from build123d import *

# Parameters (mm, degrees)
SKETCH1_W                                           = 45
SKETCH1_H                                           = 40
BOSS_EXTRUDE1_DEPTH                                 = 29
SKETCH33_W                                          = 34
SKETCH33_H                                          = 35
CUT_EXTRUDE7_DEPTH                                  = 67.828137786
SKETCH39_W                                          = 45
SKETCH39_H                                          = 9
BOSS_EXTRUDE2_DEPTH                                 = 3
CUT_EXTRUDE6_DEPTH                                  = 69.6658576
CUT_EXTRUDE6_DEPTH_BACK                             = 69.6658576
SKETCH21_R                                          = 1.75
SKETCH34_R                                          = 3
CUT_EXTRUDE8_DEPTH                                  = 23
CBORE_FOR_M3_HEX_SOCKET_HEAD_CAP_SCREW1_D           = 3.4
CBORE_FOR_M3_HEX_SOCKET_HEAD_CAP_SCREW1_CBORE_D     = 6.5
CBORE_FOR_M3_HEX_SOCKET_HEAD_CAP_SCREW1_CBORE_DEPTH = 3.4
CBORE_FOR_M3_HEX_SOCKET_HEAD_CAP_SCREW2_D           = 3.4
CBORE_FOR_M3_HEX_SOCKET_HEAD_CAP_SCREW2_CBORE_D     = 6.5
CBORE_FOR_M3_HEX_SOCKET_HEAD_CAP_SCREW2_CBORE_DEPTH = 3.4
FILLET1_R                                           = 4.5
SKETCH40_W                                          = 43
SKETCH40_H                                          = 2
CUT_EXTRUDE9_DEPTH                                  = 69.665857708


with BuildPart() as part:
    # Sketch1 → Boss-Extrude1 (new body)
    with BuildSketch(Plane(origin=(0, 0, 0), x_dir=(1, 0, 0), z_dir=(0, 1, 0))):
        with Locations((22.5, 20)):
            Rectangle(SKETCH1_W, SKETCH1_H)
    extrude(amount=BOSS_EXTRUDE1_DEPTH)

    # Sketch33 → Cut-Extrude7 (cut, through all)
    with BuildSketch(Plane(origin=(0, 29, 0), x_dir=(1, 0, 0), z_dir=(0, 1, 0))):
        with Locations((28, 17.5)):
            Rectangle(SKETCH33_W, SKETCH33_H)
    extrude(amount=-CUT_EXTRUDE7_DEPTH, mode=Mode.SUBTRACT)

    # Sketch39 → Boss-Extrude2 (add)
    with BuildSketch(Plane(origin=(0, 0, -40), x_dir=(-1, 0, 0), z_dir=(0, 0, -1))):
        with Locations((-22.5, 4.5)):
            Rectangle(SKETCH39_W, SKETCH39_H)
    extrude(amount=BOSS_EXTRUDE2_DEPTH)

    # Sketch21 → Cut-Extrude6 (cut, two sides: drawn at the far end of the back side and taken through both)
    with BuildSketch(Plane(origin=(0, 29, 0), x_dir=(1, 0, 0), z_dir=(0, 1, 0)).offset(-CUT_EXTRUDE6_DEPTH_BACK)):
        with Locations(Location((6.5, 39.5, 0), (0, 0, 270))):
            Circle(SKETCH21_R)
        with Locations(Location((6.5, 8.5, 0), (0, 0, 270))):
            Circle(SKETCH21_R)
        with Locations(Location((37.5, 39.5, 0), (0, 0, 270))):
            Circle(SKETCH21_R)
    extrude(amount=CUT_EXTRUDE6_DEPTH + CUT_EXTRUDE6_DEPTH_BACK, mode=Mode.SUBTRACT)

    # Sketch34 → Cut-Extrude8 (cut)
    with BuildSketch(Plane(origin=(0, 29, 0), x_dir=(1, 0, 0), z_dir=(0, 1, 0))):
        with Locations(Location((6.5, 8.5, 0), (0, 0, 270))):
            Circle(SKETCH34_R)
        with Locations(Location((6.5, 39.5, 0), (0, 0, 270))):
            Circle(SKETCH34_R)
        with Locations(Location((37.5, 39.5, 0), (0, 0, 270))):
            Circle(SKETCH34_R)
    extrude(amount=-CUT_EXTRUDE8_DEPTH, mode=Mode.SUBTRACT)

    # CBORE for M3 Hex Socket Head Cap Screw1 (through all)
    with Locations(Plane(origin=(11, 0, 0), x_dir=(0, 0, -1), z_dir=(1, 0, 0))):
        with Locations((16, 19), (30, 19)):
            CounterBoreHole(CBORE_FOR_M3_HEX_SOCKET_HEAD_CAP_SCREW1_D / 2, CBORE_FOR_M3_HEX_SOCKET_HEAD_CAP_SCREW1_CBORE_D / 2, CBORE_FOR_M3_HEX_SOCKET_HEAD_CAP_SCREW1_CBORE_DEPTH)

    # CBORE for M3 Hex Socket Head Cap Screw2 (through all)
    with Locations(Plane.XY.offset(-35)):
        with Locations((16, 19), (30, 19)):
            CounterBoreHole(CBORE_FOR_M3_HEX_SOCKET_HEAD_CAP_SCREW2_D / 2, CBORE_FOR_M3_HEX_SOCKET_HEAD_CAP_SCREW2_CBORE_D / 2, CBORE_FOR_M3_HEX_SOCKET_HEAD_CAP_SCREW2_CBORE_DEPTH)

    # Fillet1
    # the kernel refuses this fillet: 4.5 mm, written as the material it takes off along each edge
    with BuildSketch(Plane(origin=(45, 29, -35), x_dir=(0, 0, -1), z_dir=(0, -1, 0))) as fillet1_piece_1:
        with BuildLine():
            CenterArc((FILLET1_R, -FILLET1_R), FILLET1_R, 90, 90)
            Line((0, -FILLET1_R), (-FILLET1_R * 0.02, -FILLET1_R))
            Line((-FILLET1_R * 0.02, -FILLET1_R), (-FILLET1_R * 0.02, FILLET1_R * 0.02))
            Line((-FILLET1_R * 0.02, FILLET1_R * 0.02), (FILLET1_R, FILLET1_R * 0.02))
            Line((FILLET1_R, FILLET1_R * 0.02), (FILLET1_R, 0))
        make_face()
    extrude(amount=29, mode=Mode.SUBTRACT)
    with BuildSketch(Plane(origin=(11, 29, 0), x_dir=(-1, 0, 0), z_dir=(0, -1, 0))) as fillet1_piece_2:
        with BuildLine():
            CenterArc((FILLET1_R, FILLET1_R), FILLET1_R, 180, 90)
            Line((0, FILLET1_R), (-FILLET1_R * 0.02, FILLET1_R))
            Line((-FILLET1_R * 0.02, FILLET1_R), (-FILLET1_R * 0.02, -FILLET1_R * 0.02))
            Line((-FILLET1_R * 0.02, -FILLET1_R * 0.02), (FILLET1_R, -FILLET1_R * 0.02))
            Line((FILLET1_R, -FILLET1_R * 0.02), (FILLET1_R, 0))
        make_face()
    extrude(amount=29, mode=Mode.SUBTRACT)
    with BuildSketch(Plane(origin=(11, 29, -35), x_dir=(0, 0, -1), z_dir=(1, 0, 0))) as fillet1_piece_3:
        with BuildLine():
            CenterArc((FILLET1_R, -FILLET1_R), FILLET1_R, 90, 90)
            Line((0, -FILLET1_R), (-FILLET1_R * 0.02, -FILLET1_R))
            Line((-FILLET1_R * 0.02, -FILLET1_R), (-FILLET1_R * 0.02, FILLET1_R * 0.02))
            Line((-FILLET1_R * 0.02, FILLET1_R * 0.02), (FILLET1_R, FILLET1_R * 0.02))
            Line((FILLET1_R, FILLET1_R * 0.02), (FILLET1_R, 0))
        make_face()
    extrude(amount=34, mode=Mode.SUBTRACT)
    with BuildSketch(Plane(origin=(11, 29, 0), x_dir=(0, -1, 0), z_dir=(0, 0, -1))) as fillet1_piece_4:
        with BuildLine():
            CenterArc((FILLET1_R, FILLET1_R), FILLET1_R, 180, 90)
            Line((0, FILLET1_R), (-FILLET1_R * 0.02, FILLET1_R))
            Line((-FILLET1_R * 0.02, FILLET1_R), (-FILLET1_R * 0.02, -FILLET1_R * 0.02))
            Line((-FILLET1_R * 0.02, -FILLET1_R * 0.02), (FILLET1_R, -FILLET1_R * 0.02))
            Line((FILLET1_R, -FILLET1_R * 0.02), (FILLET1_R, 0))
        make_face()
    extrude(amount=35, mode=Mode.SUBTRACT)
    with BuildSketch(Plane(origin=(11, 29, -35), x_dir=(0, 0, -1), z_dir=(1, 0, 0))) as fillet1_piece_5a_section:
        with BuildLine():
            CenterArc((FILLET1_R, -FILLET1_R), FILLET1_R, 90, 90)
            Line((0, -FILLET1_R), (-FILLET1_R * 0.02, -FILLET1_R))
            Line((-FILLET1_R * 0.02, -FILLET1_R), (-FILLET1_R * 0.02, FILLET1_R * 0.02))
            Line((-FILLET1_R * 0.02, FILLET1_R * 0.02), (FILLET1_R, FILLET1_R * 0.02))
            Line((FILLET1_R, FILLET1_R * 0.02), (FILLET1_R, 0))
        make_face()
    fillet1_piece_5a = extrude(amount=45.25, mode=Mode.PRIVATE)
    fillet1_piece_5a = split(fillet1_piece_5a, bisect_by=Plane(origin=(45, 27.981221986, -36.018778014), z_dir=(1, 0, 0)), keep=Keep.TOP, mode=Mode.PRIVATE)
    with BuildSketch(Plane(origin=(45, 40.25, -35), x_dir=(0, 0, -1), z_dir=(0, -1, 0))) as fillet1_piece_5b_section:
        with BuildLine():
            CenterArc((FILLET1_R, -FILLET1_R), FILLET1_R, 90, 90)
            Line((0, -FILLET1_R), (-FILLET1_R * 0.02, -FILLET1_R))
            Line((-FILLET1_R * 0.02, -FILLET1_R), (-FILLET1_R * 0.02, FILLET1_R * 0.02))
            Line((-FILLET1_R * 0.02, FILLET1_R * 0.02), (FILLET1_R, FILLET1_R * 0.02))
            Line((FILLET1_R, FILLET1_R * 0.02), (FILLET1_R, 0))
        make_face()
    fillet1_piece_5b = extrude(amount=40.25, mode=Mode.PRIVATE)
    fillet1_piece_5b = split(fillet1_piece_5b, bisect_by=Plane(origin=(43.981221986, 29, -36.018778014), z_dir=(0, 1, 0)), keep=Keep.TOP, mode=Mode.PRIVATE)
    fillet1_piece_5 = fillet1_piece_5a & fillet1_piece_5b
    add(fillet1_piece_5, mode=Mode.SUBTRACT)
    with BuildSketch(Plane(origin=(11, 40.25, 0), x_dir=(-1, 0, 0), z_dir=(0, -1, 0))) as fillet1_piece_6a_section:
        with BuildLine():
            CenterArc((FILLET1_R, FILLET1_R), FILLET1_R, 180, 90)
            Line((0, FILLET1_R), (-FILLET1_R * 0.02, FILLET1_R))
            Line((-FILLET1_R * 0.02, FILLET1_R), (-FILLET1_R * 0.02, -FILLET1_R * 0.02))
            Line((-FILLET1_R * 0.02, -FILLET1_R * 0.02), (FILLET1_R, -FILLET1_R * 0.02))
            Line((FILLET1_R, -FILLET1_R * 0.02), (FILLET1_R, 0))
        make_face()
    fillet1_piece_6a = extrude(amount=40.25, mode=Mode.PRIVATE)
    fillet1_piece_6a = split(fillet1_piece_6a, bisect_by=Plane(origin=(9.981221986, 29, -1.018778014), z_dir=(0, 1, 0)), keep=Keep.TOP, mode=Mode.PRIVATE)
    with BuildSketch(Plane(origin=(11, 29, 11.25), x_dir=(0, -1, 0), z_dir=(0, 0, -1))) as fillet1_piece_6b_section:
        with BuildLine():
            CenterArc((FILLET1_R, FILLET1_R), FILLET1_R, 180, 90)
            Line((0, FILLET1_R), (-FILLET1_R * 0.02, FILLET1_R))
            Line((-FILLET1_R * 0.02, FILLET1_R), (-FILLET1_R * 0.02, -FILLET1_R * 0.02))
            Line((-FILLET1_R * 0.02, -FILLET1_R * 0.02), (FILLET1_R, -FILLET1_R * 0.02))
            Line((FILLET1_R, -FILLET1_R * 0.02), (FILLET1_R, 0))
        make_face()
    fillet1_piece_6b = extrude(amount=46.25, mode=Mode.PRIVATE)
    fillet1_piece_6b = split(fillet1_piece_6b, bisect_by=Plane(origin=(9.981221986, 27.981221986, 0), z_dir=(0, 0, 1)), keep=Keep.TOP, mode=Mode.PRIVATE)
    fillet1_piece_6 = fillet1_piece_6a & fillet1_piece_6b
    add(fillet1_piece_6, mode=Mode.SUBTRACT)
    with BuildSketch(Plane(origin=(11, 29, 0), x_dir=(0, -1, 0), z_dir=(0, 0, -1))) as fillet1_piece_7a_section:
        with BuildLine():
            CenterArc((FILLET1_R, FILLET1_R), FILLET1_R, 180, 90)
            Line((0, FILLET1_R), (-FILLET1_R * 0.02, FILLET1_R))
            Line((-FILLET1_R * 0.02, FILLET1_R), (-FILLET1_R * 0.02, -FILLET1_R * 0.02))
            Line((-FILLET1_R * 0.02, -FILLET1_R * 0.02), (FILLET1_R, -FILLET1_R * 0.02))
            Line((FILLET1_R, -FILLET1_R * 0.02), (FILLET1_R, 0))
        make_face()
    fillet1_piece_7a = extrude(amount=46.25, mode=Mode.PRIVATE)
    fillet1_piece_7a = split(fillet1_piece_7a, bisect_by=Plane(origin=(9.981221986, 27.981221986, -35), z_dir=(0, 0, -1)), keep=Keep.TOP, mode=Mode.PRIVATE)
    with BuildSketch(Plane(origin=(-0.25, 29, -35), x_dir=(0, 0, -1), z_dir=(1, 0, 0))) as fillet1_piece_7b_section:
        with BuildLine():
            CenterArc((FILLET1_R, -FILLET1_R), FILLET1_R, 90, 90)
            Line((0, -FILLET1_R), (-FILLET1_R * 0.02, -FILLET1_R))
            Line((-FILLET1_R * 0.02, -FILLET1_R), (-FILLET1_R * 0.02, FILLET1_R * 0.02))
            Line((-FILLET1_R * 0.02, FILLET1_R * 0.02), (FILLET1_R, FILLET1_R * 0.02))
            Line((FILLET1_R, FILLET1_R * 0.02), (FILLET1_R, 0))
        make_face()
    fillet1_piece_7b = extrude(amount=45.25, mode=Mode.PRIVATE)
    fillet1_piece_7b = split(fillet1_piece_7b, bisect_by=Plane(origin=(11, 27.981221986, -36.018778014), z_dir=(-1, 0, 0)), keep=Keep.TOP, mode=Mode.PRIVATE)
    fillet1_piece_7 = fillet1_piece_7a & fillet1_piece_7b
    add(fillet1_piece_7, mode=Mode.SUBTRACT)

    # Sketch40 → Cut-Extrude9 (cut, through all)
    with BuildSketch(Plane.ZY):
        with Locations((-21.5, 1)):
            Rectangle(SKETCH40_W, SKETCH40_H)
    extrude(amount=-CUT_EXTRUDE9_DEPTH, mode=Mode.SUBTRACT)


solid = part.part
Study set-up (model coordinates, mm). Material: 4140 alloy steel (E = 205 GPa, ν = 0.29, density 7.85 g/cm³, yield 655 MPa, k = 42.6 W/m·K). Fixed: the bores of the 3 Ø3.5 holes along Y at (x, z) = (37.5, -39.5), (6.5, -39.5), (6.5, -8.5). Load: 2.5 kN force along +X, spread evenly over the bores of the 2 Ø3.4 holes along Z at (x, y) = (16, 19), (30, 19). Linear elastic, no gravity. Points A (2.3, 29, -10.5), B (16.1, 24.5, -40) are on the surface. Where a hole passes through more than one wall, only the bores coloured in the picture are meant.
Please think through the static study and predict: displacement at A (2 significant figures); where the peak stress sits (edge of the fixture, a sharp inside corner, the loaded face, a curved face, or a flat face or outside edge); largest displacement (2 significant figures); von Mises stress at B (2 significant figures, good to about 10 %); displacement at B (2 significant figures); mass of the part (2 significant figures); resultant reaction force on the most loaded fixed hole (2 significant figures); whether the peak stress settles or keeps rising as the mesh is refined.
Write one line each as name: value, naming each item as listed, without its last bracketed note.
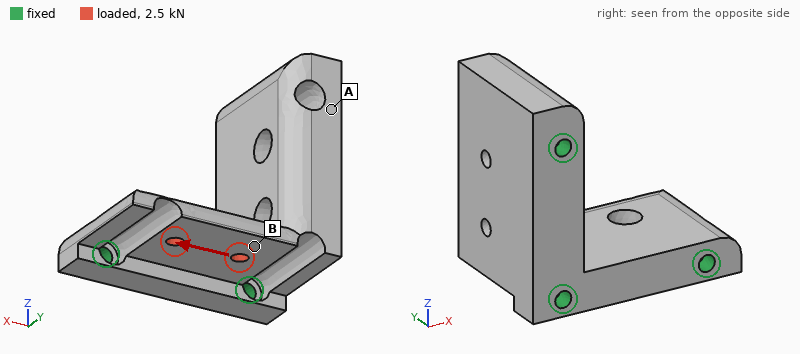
displacement at A: 3.6 µm
where the peak stress sits: edge of the fixture
largest displacement: 15 µm
von Mises stress at B: 21 MPa
displacement at B: 7.1 µm
mass of the part: 120 g
resultant reaction force on the most loaded fixed hole: 1.6 kN
whether the peak stress settles or keeps rising as the mesh is refined: keeps rising
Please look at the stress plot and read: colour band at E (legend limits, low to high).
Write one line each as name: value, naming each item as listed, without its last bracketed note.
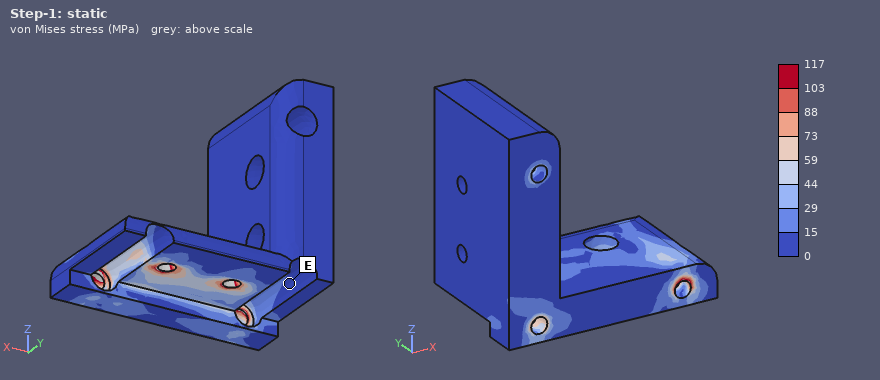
colour band at E: 0 to 15 MPa
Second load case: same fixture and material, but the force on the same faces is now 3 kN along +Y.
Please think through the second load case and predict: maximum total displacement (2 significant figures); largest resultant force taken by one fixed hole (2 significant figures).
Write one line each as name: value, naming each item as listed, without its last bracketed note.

maximum total displacement: 12 µm
largest resultant force taken by one fixed hole: 1.7 kN
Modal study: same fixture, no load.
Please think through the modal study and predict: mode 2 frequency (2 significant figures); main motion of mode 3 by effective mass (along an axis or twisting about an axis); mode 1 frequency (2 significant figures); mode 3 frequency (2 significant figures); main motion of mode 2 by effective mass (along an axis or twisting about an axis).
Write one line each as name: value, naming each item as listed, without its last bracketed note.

mode 2 frequency: 9000 Hz
main motion of mode 3 by effective mass: along Z
mode 1 frequency: 8100 Hz
mode 3 frequency: 15 kHz
main motion of mode 2 by effective mass: along X
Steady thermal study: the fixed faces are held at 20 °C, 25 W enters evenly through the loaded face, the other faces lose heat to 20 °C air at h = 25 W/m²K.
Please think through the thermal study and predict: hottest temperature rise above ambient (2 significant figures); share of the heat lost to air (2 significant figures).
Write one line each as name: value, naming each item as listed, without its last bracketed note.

hottest temperature rise above ambient: 86 K
share of the heat lost to air: 13 %
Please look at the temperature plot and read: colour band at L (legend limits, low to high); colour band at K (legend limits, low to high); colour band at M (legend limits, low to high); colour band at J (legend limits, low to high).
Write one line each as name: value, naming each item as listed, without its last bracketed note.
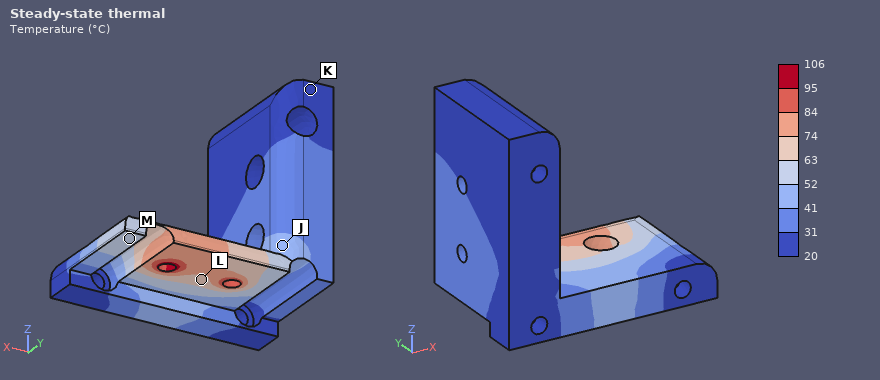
colour band at L: 63 to 74 °C
colour band at K: 20 to 31 °C
colour band at M: 52 to 63 °C
colour band at J: 41 to 52 °C
